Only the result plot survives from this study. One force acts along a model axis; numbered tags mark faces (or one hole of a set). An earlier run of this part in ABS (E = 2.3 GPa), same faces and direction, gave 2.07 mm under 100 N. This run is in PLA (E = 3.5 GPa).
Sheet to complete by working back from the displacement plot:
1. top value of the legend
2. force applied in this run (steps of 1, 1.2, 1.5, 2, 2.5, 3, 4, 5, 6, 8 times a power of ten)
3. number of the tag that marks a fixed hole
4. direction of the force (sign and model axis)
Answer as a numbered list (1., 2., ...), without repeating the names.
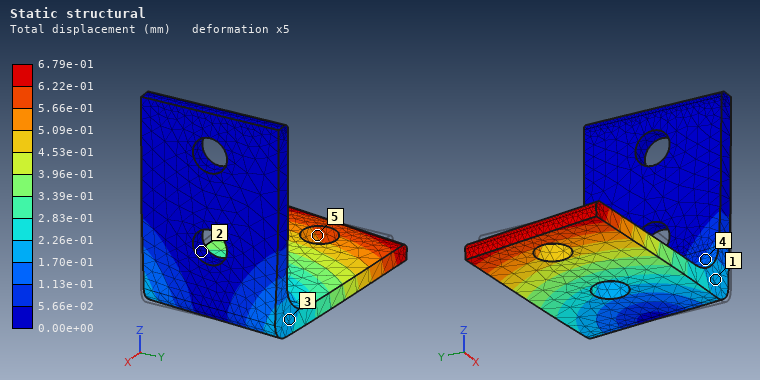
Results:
1. 6.79e-01 mm
2. 50 N
3. 2
4. +Y
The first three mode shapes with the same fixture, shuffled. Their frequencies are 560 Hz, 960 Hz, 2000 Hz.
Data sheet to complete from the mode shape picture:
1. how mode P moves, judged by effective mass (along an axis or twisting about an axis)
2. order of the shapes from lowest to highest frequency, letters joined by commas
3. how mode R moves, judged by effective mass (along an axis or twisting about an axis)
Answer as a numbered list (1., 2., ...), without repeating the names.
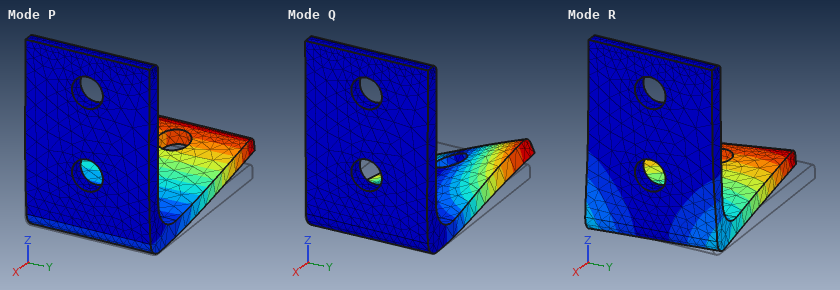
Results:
1. along Z
2. P, R, Q
3. along Y
